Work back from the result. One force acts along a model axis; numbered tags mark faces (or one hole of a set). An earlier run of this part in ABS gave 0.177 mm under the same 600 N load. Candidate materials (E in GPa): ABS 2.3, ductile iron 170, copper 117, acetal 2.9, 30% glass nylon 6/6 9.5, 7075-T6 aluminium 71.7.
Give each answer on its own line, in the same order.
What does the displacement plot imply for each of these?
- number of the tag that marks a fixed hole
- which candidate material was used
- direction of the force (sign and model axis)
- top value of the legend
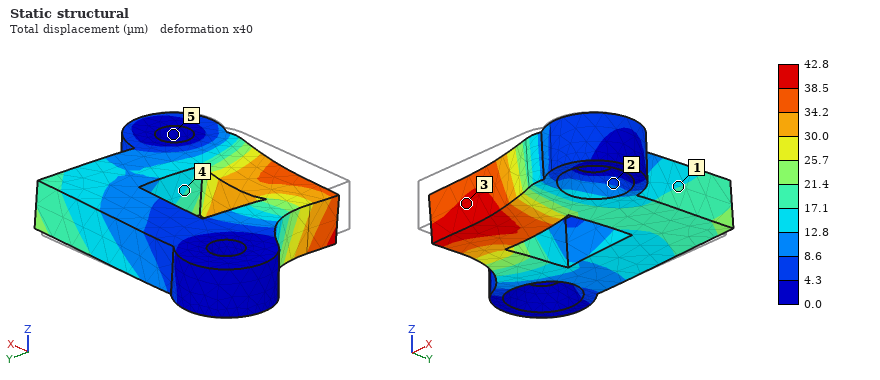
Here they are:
5
30% glass nylon 6/6
+Y
42.8 µm
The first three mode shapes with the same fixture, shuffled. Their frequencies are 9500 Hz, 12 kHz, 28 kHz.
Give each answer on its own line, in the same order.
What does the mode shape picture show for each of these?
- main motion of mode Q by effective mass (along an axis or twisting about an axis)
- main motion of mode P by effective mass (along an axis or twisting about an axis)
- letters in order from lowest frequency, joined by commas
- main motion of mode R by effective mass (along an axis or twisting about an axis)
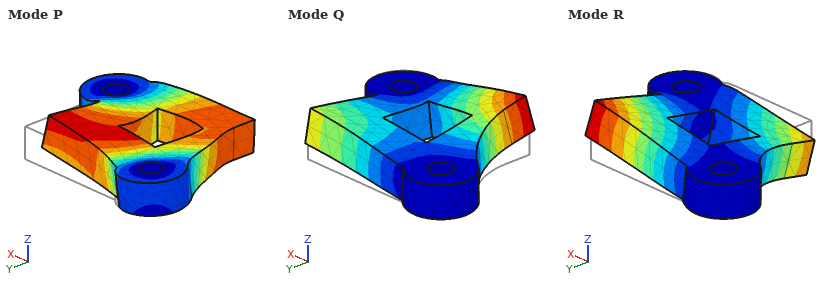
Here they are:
along Z
along Y
R, Q, P
twisting about X
